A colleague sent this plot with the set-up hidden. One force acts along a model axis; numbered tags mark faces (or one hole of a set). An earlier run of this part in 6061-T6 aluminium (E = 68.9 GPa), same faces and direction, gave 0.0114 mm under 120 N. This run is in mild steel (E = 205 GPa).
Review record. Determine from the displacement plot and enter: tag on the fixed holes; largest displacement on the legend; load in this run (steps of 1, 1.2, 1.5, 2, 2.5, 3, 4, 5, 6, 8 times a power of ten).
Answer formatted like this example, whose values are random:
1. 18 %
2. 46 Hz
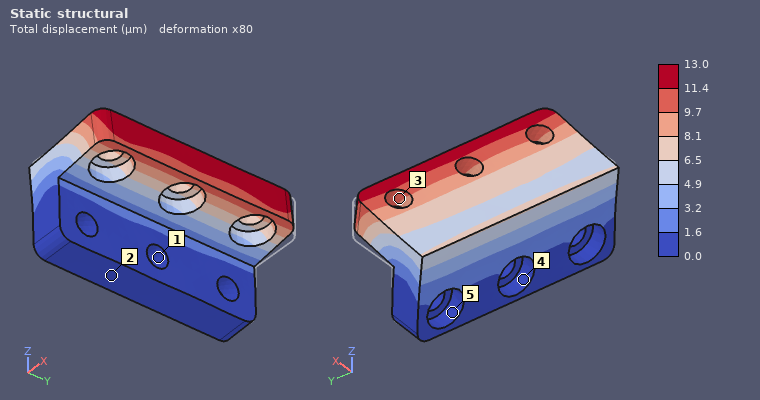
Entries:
1. 1
2. 13.0 µm
3. 400 N
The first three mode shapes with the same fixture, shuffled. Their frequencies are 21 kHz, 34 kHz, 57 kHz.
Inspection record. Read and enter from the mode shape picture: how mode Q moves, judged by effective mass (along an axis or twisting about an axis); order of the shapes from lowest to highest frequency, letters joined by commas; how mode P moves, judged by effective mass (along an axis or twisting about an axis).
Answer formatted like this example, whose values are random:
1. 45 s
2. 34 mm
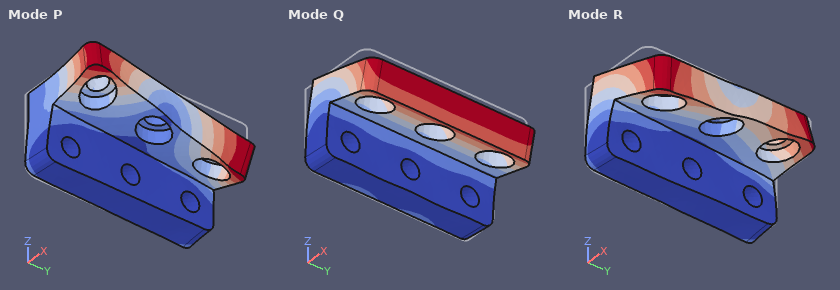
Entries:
1. along X
2. Q, R, P
3. along Y
